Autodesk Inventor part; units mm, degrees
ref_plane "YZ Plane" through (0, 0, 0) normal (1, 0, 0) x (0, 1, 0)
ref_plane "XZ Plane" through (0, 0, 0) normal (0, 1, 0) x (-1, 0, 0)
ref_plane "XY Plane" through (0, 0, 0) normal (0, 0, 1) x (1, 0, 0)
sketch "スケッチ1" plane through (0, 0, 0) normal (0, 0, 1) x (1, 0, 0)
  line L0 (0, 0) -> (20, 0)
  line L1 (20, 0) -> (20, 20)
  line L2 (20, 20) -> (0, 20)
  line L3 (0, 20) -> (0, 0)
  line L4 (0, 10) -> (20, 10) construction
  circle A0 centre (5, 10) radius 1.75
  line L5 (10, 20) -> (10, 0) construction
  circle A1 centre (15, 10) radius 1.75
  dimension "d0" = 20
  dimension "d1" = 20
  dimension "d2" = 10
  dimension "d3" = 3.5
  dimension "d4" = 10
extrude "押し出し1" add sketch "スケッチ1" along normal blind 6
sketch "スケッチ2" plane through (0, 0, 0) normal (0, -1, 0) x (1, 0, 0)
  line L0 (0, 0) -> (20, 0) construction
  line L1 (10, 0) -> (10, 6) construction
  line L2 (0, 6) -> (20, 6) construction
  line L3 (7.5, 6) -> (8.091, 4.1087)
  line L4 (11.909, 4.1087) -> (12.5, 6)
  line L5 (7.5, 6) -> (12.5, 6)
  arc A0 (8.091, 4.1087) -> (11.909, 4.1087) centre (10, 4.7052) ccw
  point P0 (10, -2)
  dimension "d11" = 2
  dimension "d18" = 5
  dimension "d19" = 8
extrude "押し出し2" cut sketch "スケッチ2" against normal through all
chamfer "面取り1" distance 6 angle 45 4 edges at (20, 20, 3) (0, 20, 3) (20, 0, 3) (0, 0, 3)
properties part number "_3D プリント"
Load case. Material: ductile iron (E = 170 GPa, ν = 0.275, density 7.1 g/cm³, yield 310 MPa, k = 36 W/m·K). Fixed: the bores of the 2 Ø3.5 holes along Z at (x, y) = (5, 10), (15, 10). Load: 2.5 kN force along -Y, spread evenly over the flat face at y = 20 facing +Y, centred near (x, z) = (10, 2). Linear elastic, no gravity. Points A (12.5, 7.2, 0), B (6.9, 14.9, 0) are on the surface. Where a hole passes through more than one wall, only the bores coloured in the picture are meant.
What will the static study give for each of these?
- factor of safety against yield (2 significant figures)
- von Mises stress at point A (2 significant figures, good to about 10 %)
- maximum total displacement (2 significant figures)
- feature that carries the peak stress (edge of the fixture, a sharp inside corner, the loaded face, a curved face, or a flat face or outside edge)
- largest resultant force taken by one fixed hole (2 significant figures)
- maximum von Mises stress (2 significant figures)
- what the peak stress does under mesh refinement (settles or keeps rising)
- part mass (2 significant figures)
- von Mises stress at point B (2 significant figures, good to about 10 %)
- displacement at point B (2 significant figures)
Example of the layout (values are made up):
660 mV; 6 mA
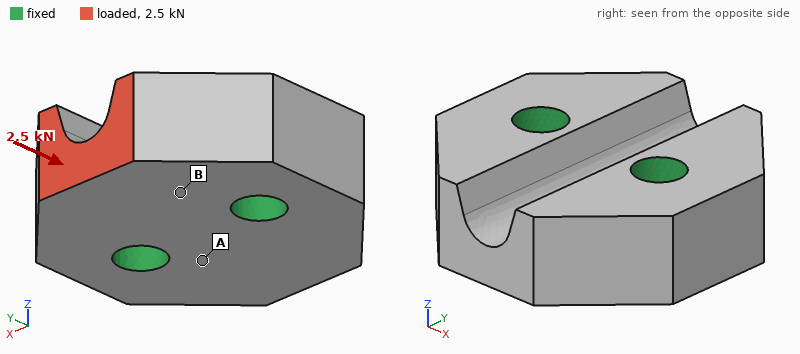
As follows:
3.0; 12 MPa; 4.0 µm; the loaded face; 1.3 kN; 100 MPa; settles; 11 g; 58 MPa; 1.4 µm
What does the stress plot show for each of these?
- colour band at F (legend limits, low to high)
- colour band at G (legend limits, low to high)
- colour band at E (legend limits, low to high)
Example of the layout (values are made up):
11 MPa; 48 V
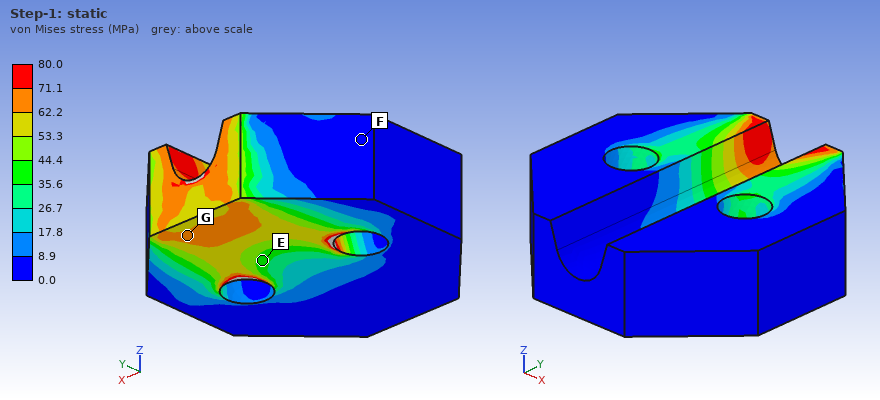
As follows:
0.0 to 8.9 MPa; 62.2 to 71.1 MPa; 35.6 to 44.4 MPa
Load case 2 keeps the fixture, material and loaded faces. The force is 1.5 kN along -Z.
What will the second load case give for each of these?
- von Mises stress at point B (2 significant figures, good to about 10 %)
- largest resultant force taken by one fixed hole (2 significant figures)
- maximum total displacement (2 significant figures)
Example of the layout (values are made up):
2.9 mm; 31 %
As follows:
110 MPa; 750 N; 17 µm
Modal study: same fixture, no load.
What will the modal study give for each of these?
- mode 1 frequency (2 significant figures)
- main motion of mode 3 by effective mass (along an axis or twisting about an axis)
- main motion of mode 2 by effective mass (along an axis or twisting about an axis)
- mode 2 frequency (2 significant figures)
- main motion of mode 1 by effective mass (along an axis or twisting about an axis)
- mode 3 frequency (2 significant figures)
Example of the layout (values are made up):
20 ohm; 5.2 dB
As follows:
51 kHz; twisting about Z; along Z; 55 kHz; twisting about X; 65 kHz
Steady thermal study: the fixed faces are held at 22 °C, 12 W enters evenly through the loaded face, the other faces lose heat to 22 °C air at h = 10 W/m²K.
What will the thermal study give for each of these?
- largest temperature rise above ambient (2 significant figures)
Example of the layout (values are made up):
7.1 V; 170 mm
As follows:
53 K
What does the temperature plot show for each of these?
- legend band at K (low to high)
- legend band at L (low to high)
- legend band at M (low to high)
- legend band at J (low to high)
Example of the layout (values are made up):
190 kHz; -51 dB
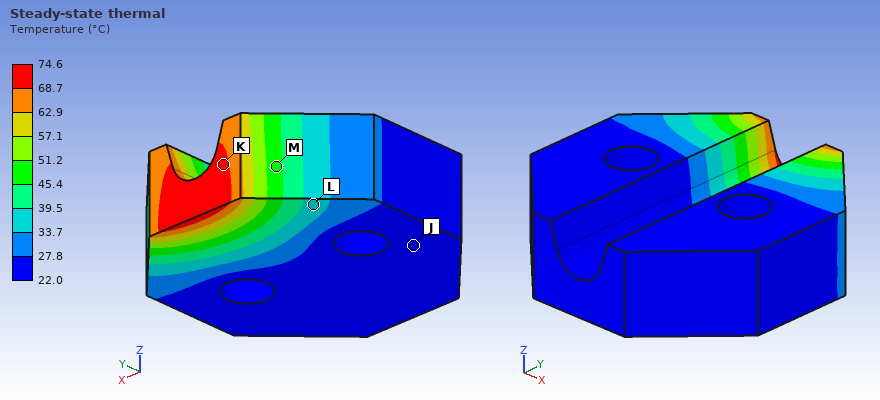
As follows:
68.7 to 74.6 °C; 33.7 to 39.5 °C; 45.4 to 51.2 °C; 22.0 to 27.8 °C
